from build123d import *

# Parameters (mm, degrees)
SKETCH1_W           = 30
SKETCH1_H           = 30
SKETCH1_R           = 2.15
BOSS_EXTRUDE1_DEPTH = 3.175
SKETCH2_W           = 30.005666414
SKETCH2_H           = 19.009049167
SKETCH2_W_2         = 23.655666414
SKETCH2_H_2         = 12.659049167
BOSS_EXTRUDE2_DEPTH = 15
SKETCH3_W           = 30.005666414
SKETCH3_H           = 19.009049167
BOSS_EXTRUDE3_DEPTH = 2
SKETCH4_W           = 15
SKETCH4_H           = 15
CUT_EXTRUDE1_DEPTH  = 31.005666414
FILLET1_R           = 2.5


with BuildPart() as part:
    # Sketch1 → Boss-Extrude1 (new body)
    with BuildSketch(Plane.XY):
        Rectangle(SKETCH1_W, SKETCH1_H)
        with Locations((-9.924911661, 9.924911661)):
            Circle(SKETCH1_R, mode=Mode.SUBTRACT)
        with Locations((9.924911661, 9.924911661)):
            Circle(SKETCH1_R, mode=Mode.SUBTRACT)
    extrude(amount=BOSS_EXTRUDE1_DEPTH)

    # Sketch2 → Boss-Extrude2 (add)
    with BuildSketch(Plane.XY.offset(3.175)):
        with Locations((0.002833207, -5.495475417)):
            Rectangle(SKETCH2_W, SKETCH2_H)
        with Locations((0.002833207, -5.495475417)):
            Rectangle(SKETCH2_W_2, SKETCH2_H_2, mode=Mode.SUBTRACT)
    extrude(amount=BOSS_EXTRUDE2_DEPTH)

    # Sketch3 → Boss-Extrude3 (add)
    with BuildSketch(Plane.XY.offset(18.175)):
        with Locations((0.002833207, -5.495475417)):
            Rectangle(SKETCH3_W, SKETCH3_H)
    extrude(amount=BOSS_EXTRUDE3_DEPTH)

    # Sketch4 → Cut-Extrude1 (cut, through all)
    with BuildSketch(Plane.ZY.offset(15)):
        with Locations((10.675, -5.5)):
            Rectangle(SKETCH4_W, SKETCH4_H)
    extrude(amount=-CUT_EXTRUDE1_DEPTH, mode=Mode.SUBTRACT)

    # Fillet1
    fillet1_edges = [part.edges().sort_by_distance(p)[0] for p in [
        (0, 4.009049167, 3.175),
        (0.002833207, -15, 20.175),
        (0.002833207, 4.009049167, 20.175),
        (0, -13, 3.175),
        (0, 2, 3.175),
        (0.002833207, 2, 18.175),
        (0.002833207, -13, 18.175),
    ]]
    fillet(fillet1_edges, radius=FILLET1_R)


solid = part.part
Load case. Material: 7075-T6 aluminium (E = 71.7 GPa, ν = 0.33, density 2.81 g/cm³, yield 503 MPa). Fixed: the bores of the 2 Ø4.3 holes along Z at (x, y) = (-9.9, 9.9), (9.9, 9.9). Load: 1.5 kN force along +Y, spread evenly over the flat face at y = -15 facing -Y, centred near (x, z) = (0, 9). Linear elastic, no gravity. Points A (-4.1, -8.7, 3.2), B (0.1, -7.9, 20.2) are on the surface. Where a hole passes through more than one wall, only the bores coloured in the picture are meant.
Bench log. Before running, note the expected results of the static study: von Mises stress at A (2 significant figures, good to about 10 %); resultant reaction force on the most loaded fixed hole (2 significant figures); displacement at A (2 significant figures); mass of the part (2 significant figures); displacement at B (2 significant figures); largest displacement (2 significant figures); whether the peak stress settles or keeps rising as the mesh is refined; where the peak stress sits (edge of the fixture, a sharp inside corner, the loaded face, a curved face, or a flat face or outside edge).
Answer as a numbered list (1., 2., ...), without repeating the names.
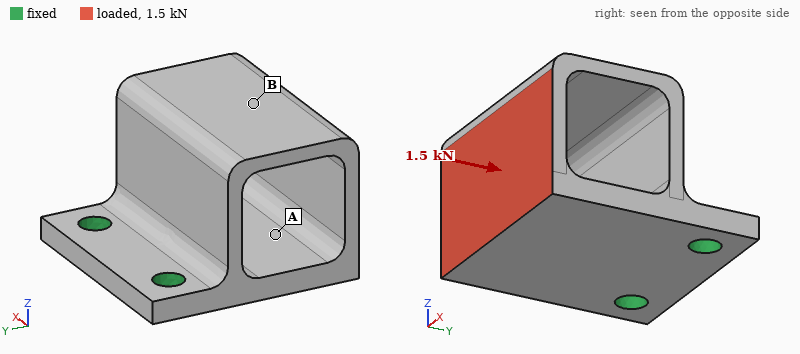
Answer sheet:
1. 84 MPa
2. 760 N
3. 0.19 mm
4. 16 g
5. 0.39 mm
6. 0.43 mm
7. keeps rising
8. edge of the fixture
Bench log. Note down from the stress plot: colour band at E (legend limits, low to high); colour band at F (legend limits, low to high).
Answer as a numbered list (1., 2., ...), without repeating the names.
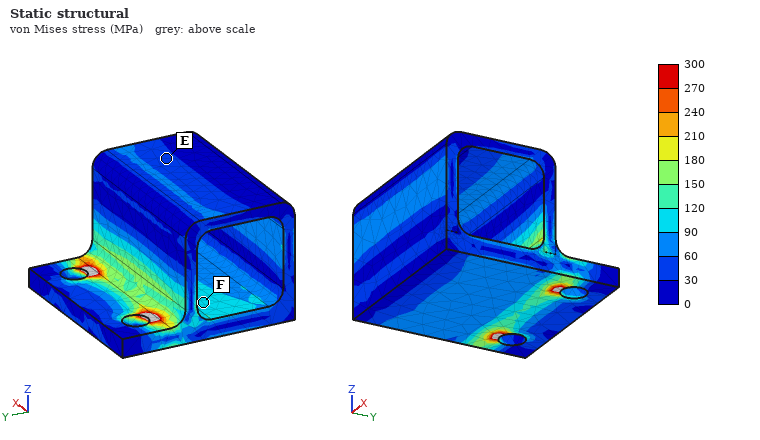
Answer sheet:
1. 30 to 60 MPa
2. 90 to 120 MPa
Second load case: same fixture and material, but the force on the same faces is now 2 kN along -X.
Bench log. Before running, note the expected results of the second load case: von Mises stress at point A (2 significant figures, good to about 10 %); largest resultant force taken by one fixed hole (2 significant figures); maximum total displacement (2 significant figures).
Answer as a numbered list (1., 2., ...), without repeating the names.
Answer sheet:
1. 78 MPa
2. 2.5 kN
3. 0.17 mm
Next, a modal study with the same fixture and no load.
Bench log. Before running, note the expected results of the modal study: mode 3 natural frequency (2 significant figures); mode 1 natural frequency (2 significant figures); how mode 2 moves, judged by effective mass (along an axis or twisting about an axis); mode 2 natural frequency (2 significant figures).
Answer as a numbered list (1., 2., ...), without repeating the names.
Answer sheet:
1. 8300 Hz
2. 2200 Hz
3. along X
4. 6600 Hz
